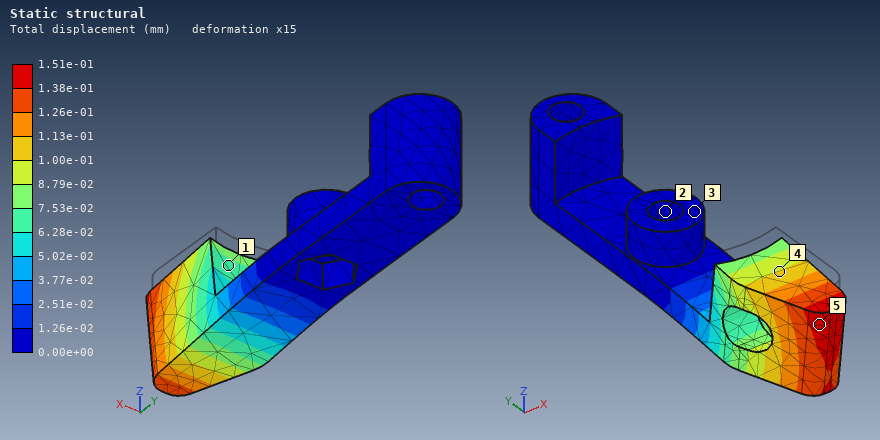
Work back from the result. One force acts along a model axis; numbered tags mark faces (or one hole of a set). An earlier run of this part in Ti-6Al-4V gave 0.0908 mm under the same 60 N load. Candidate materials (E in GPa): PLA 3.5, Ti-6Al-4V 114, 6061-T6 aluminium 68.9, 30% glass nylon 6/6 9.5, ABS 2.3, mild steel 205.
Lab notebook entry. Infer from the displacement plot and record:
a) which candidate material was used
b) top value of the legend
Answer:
6061-T6 aluminium
1.51e-01 mm
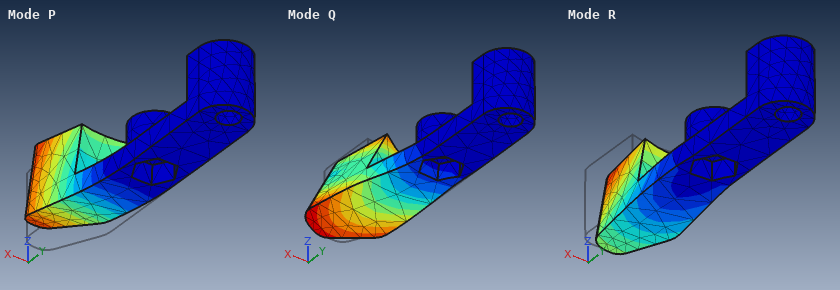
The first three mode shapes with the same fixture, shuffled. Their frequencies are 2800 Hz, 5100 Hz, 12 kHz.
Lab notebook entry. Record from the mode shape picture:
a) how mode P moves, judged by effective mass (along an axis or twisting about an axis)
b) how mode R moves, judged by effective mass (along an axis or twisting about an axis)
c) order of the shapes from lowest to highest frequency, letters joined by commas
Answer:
along Z
along X
P, R, Q
